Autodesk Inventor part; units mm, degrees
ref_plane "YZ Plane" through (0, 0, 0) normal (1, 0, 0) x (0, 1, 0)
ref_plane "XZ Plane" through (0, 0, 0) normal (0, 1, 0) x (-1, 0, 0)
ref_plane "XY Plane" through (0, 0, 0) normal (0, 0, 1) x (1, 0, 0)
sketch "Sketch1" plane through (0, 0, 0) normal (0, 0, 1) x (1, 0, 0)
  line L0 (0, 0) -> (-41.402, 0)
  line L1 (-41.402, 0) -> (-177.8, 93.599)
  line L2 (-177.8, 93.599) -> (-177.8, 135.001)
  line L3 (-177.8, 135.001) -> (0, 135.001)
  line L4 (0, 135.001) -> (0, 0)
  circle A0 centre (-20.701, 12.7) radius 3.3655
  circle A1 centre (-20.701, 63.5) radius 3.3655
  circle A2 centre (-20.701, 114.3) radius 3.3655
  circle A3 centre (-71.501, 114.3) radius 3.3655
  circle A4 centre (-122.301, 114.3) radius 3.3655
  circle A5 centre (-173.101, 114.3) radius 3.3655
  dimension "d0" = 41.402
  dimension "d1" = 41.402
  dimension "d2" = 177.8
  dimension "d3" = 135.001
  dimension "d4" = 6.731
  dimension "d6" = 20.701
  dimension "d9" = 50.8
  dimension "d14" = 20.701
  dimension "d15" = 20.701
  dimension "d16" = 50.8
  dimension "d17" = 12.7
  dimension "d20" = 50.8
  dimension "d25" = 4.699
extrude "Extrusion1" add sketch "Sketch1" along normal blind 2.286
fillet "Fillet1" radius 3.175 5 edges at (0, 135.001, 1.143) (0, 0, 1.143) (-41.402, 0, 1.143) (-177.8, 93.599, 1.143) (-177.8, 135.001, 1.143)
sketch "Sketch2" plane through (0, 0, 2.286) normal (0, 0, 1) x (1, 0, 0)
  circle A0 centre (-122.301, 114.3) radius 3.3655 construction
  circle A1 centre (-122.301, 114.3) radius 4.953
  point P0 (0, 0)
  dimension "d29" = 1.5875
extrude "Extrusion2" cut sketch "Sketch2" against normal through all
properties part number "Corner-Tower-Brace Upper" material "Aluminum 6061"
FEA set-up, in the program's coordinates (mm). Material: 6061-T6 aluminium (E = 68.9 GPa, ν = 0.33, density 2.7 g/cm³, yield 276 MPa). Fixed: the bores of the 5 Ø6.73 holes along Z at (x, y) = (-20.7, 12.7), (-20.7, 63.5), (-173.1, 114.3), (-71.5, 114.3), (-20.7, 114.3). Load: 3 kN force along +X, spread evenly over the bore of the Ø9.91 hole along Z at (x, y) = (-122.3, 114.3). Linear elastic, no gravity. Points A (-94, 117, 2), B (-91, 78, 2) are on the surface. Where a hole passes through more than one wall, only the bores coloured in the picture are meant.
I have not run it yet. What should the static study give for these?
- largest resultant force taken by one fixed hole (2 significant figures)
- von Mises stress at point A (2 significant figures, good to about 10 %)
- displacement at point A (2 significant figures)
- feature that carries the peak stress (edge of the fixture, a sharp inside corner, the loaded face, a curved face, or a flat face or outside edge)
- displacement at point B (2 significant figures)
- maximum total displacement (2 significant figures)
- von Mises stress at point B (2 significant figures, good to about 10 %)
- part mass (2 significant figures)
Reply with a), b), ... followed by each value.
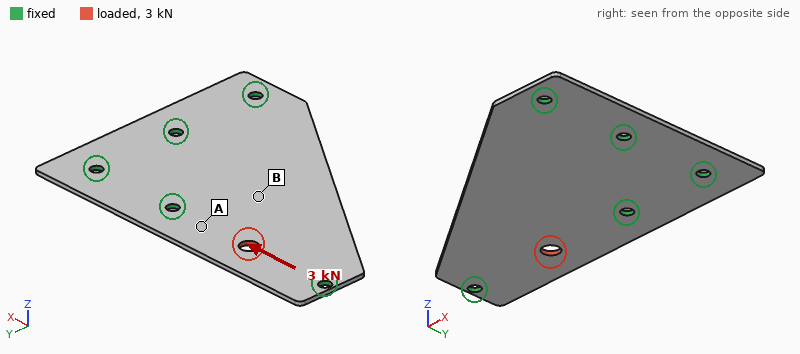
a) 1.2 kN
b) 21 MPa
c) 7.2 µm
d) the loaded face
e) 4.2 µm
f) 18 µm
g) 4.5 MPa
h) 110 g
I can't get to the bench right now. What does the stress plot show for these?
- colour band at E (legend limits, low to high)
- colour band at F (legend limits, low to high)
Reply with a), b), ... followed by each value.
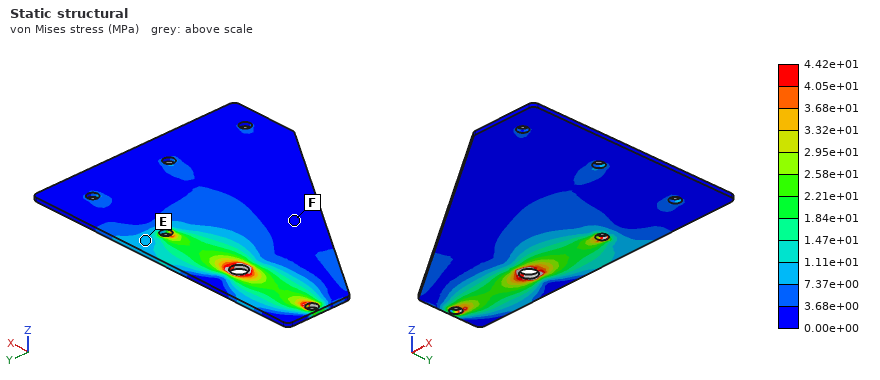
a) 7.37e+00 to 1.11e+01 MPa
b) 0.00e+00 to 3.68e+00 MPa
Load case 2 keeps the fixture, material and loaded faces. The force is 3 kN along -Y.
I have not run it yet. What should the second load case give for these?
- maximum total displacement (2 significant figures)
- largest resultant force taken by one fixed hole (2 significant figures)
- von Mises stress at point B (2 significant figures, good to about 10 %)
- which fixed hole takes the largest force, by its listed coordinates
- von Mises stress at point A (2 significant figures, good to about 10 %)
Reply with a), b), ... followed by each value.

a) 39 µm
b) 1.6 kN
c) 17 MPa
d) (-71.5, 114.3)
e) 18 MPa
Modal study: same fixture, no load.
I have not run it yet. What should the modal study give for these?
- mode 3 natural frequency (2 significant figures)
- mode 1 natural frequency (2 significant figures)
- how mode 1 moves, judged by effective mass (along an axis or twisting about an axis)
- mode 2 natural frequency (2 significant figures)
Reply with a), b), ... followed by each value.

a) 1400 Hz
b) 550 Hz
c) along Z
d) 1100 Hz
